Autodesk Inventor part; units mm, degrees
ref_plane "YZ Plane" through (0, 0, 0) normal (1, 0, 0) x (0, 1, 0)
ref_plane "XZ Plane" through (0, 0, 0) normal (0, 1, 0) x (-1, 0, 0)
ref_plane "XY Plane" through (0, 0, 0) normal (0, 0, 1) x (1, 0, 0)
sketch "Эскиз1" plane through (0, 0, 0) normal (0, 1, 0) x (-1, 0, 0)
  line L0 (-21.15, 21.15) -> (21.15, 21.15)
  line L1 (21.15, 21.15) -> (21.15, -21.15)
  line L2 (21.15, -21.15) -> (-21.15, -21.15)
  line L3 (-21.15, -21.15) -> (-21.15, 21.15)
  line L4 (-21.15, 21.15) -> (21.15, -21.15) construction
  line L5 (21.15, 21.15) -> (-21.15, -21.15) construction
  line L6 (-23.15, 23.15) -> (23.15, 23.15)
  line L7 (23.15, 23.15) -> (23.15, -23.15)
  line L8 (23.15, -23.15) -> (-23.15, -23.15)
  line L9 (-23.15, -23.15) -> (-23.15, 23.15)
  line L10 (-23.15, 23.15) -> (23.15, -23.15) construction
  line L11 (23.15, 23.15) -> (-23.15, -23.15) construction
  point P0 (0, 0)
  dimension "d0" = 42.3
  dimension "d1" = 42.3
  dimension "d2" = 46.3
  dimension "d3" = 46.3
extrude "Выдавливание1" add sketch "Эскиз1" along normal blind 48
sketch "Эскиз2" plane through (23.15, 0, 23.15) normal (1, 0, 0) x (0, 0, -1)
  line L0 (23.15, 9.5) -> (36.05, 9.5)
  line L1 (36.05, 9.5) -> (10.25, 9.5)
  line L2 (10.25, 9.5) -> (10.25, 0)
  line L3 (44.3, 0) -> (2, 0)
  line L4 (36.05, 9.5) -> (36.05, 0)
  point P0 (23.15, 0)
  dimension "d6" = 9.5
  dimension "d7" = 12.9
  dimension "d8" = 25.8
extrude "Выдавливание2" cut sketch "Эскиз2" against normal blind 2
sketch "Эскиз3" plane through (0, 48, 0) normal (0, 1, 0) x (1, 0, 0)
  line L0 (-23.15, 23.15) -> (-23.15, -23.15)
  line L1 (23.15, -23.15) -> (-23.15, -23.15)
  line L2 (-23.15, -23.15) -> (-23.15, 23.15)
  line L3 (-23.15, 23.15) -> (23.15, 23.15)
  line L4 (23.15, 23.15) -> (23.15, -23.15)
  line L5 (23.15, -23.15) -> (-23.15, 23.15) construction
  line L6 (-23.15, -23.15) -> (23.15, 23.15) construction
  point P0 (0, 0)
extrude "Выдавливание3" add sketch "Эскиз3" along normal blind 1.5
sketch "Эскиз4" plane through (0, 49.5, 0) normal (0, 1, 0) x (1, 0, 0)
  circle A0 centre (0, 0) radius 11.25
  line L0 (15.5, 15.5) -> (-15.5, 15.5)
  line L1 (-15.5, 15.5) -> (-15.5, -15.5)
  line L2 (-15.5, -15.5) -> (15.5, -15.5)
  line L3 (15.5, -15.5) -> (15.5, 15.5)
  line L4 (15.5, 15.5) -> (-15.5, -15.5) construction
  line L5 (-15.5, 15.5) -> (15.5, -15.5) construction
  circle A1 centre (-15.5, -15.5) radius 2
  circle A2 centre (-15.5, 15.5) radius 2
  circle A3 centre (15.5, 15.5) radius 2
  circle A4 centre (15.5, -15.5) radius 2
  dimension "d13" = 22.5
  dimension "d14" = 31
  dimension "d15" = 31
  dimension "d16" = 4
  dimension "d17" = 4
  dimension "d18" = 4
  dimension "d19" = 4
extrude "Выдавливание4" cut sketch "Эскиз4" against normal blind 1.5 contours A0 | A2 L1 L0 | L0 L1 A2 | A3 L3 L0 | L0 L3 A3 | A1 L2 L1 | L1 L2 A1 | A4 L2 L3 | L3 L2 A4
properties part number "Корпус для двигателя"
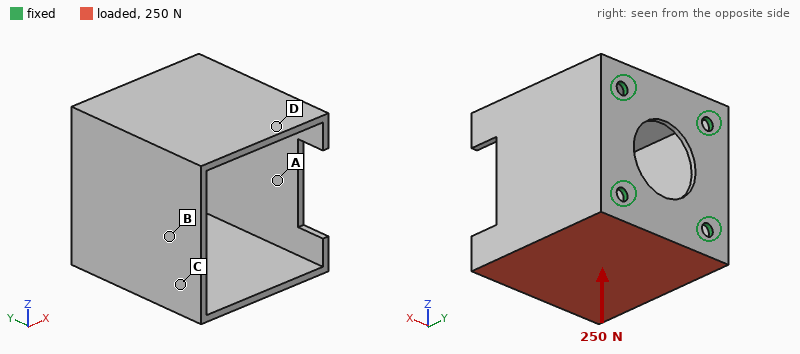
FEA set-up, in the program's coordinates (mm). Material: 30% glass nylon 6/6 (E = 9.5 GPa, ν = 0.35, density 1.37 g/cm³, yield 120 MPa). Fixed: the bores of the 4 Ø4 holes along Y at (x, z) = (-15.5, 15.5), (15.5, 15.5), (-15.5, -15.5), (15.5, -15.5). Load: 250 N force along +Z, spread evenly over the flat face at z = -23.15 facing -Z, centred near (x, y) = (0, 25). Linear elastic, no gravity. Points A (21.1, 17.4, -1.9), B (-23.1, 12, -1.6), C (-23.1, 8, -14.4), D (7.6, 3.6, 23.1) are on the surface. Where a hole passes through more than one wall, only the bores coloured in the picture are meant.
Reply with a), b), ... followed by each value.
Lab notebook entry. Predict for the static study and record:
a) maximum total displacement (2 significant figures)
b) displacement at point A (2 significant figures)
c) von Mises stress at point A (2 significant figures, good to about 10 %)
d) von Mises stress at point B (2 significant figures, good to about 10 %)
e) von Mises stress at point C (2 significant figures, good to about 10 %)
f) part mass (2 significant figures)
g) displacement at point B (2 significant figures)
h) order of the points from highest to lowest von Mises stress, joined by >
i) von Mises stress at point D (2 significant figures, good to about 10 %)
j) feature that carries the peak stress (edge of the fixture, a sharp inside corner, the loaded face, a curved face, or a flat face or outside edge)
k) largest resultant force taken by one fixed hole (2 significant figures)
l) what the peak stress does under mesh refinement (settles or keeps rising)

a) 0.54 mm
b) 0.14 mm
c) 6.5 MPa
d) 4.3 MPa
e) 10 MPa
f) 26 g
g) 0.15 mm
h) C > A > B > D
i) 2.0 MPa
j) edge of the fixture
k) 130 N
l) keeps rising
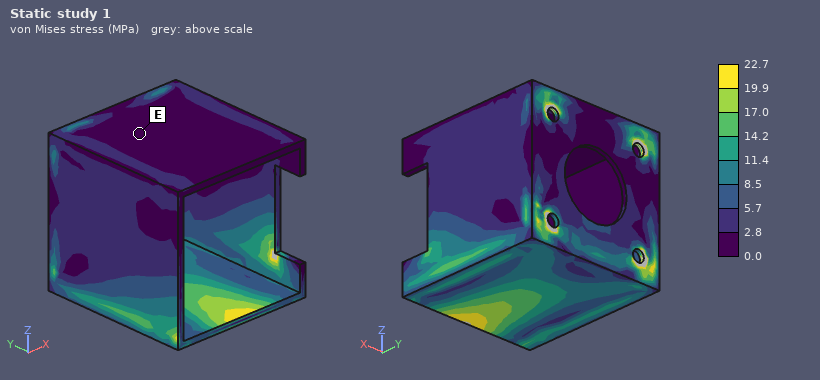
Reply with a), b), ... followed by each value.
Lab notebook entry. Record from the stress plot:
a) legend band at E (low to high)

a) 0.0 to 2.8 MPa
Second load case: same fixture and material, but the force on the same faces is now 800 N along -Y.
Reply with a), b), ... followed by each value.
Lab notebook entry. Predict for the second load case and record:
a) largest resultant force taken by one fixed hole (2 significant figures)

a) 460 N
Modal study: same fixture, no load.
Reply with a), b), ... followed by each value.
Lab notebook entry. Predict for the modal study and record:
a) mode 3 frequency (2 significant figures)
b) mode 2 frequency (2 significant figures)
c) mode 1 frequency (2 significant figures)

a) 1600 Hz
b) 1500 Hz
c) 1500 Hz
